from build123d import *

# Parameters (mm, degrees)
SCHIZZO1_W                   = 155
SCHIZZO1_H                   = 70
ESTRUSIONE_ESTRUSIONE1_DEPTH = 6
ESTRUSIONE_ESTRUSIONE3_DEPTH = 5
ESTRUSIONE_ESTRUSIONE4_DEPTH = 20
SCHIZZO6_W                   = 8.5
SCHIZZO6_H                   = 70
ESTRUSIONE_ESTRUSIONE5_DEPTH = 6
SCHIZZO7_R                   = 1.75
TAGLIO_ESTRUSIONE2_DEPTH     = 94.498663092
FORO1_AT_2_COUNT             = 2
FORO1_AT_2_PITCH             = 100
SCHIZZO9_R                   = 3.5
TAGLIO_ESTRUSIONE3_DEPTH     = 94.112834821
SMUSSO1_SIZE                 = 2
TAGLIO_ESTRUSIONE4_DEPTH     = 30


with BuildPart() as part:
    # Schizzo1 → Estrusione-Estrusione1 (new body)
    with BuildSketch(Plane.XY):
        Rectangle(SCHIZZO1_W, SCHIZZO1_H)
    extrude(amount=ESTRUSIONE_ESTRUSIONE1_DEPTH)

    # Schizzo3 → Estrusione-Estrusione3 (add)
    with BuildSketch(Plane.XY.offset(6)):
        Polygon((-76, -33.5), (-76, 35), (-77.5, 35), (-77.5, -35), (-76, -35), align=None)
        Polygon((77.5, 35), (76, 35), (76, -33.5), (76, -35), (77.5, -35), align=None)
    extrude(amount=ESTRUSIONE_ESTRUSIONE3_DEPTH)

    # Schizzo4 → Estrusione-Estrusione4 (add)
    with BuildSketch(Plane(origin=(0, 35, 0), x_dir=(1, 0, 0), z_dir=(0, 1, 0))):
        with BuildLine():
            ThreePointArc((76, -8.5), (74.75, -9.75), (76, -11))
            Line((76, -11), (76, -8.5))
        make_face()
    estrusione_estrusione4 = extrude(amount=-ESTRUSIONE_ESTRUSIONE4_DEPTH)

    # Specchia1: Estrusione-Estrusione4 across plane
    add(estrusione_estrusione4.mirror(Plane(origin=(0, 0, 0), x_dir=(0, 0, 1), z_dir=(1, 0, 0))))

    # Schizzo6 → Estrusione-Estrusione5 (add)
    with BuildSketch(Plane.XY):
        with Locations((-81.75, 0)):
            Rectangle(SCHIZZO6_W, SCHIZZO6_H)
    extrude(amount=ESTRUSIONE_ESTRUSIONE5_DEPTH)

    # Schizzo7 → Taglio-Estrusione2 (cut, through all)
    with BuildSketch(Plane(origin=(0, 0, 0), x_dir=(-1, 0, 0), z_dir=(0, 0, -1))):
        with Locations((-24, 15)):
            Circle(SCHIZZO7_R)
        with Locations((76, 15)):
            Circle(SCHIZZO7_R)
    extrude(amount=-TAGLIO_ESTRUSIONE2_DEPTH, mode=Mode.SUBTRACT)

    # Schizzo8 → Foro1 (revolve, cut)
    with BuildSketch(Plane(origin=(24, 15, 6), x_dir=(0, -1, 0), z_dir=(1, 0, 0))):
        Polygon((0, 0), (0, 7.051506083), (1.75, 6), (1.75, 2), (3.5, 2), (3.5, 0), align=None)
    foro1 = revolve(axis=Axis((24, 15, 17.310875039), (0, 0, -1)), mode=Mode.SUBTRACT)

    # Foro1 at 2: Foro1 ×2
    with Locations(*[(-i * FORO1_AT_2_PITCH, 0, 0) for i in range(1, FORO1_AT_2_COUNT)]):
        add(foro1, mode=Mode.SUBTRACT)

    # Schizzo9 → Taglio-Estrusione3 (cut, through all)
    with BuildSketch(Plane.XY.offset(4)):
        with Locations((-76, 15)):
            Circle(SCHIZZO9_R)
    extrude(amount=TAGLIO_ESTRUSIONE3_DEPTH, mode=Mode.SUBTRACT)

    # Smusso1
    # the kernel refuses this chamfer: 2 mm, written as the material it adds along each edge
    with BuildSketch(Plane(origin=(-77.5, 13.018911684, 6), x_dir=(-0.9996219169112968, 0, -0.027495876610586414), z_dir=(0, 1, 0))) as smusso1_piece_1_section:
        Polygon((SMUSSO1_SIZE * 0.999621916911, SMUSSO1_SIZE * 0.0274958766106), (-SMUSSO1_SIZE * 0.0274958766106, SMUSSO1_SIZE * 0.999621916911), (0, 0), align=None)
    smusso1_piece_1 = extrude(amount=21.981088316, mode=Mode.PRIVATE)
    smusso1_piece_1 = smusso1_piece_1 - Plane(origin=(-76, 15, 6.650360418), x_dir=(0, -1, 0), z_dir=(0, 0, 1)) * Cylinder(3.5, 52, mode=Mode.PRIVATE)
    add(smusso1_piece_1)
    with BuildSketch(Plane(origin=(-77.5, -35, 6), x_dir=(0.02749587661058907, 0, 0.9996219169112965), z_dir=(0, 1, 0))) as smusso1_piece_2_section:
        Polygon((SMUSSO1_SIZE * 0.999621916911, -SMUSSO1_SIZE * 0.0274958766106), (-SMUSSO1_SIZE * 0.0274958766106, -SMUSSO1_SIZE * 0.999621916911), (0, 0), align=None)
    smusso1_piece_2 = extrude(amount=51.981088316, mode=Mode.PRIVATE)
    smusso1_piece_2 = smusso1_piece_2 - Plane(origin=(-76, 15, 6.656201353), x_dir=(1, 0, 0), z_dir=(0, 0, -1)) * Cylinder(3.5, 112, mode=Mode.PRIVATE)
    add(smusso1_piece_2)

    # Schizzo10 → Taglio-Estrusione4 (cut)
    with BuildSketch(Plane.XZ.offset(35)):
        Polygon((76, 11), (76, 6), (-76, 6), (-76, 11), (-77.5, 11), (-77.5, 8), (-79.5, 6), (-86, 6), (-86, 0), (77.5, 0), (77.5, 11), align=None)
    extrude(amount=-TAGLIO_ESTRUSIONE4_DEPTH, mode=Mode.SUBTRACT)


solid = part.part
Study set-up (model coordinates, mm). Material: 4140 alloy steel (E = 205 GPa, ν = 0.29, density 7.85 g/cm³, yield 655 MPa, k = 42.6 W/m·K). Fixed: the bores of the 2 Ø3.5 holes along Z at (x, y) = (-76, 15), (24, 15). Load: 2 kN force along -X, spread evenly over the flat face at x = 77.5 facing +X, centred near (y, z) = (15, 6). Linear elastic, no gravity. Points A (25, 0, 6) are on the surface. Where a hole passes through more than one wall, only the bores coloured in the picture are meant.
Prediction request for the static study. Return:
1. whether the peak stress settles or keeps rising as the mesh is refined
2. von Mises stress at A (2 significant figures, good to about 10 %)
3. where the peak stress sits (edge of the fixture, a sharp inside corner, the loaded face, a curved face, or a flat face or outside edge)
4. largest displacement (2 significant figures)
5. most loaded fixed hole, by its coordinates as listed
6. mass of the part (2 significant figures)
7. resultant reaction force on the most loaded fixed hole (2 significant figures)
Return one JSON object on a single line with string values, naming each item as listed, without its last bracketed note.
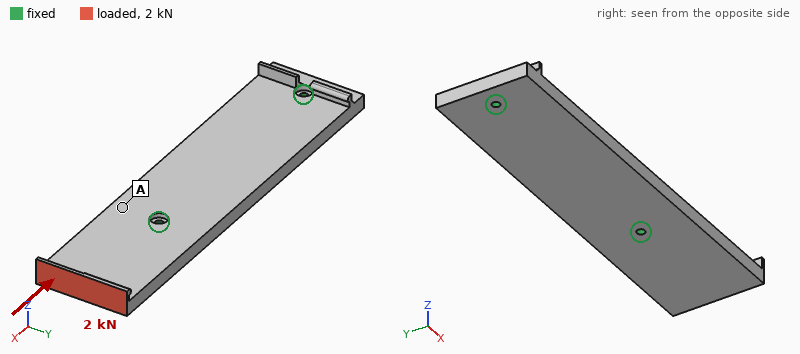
{"whether the peak stress settles or keeps rising as the mesh is refined": "keeps rising", "von Mises stress at A": "22 MPa", "where the peak stress sits": "edge of the fixture", "largest displacement": "80 µm", "most loaded fixed hole, by its coordinates as listed": "(24, 15)", "mass of the part": "310 g", "resultant reaction force on the most loaded fixed hole": "1.5 kN"}
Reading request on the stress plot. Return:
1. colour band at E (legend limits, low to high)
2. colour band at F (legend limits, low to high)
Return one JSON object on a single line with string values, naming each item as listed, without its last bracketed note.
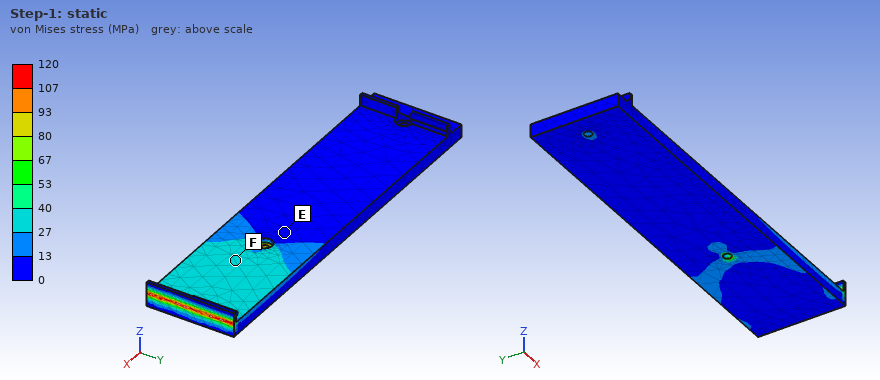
{"colour band at E": "0 to 13 MPa", "colour band at F": "27 to 40 MPa"}
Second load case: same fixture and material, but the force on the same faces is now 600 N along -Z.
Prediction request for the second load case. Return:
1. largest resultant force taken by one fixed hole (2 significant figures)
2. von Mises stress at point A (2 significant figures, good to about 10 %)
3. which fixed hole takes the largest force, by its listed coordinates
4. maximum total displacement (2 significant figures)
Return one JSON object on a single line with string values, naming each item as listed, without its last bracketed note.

{"largest resultant force taken by one fixed hole": "1.1 kN", "von Mises stress at point A": "92 MPa", "which fixed hole takes the largest force, by its listed coordinates": "(24, 15)", "maximum total displacement": "0.32 mm"}
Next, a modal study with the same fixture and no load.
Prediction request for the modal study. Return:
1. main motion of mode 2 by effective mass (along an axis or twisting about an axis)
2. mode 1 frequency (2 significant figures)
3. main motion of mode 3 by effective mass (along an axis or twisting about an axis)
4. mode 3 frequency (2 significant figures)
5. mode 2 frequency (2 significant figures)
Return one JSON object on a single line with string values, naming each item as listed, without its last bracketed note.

{"main motion of mode 2 by effective mass": "along Z", "mode 1 frequency": "1200 Hz", "main motion of mode 3 by effective mass": "twisting about X", "mode 3 frequency": "2700 Hz", "mode 2 frequency": "2400 Hz"}
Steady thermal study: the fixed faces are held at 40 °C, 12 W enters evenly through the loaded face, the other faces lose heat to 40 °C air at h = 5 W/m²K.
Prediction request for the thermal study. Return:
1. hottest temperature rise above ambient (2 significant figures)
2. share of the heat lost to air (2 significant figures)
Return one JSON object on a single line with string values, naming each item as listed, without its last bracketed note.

{"hottest temperature rise above ambient": "77 K", "share of the heat lost to air": "11 %"}
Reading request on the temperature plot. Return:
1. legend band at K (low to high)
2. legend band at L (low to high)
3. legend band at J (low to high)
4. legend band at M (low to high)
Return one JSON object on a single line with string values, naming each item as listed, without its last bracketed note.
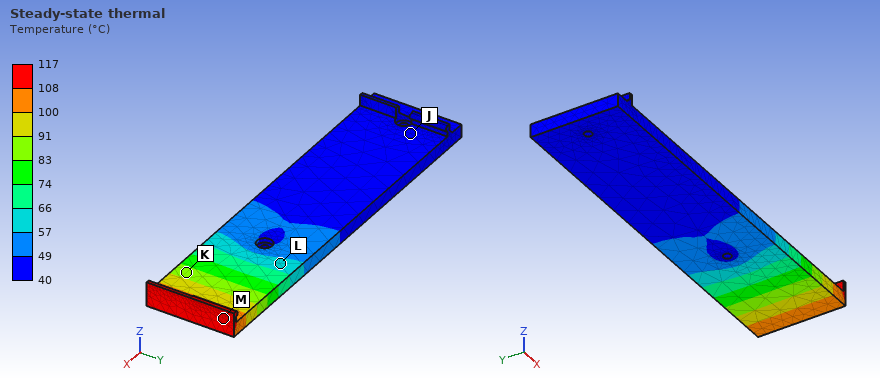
{"legend band at K": "83 to 91 °C", "legend band at L": "57 to 66 °C", "legend band at J": "40 to 49 °C", "legend band at M": "108 to 117 °C"}
